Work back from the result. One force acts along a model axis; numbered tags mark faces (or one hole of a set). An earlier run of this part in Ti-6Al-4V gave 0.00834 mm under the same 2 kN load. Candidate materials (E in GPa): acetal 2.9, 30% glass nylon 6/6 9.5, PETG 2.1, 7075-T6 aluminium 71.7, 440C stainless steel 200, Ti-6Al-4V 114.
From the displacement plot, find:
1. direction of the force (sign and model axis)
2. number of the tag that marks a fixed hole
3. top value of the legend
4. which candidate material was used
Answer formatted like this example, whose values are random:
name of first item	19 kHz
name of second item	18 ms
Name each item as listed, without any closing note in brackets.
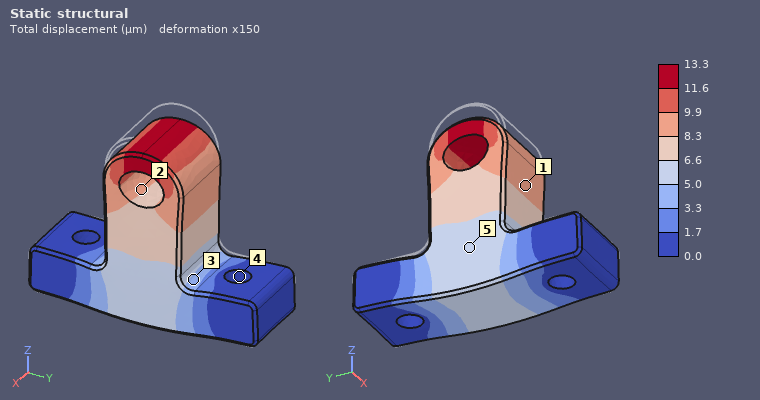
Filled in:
direction of the force	-Z
number of the tag that marks a fixed hole	4
top value of the legend	13.3 µm
which candidate material was used	7075-T6 aluminium
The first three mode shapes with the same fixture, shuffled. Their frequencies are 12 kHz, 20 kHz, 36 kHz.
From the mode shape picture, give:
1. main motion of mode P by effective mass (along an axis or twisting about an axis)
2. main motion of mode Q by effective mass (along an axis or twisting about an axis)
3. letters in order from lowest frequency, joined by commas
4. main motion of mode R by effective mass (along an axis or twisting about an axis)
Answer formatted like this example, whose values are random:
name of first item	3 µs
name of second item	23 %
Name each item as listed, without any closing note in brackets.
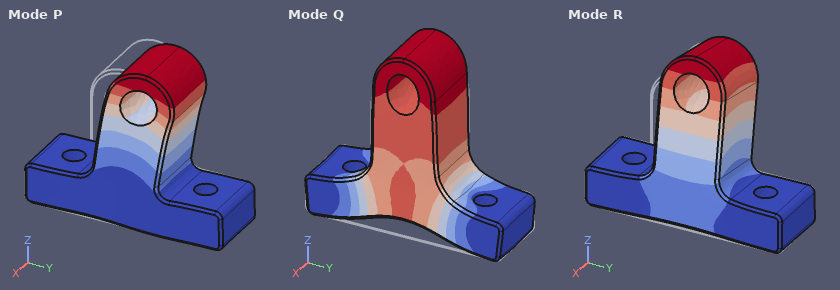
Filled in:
main motion of mode P by effective mass	along Y
main motion of mode Q by effective mass	along Z
letters in order from lowest frequency, joined by commas	R, P, Q
main motion of mode R by effective mass	along X
